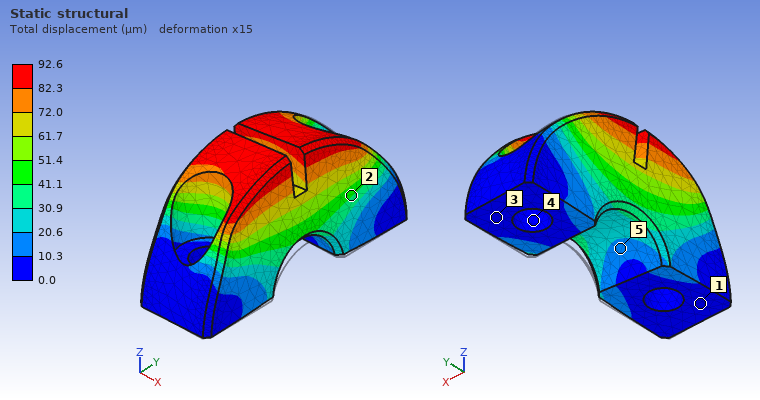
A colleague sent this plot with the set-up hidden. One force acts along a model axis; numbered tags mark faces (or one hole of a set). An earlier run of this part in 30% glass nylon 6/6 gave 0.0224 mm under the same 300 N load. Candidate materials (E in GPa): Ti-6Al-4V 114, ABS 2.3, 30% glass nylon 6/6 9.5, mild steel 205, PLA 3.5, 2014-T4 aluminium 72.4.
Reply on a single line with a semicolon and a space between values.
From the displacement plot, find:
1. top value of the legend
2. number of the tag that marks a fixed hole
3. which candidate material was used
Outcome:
92.6 µm; 4; ABS
